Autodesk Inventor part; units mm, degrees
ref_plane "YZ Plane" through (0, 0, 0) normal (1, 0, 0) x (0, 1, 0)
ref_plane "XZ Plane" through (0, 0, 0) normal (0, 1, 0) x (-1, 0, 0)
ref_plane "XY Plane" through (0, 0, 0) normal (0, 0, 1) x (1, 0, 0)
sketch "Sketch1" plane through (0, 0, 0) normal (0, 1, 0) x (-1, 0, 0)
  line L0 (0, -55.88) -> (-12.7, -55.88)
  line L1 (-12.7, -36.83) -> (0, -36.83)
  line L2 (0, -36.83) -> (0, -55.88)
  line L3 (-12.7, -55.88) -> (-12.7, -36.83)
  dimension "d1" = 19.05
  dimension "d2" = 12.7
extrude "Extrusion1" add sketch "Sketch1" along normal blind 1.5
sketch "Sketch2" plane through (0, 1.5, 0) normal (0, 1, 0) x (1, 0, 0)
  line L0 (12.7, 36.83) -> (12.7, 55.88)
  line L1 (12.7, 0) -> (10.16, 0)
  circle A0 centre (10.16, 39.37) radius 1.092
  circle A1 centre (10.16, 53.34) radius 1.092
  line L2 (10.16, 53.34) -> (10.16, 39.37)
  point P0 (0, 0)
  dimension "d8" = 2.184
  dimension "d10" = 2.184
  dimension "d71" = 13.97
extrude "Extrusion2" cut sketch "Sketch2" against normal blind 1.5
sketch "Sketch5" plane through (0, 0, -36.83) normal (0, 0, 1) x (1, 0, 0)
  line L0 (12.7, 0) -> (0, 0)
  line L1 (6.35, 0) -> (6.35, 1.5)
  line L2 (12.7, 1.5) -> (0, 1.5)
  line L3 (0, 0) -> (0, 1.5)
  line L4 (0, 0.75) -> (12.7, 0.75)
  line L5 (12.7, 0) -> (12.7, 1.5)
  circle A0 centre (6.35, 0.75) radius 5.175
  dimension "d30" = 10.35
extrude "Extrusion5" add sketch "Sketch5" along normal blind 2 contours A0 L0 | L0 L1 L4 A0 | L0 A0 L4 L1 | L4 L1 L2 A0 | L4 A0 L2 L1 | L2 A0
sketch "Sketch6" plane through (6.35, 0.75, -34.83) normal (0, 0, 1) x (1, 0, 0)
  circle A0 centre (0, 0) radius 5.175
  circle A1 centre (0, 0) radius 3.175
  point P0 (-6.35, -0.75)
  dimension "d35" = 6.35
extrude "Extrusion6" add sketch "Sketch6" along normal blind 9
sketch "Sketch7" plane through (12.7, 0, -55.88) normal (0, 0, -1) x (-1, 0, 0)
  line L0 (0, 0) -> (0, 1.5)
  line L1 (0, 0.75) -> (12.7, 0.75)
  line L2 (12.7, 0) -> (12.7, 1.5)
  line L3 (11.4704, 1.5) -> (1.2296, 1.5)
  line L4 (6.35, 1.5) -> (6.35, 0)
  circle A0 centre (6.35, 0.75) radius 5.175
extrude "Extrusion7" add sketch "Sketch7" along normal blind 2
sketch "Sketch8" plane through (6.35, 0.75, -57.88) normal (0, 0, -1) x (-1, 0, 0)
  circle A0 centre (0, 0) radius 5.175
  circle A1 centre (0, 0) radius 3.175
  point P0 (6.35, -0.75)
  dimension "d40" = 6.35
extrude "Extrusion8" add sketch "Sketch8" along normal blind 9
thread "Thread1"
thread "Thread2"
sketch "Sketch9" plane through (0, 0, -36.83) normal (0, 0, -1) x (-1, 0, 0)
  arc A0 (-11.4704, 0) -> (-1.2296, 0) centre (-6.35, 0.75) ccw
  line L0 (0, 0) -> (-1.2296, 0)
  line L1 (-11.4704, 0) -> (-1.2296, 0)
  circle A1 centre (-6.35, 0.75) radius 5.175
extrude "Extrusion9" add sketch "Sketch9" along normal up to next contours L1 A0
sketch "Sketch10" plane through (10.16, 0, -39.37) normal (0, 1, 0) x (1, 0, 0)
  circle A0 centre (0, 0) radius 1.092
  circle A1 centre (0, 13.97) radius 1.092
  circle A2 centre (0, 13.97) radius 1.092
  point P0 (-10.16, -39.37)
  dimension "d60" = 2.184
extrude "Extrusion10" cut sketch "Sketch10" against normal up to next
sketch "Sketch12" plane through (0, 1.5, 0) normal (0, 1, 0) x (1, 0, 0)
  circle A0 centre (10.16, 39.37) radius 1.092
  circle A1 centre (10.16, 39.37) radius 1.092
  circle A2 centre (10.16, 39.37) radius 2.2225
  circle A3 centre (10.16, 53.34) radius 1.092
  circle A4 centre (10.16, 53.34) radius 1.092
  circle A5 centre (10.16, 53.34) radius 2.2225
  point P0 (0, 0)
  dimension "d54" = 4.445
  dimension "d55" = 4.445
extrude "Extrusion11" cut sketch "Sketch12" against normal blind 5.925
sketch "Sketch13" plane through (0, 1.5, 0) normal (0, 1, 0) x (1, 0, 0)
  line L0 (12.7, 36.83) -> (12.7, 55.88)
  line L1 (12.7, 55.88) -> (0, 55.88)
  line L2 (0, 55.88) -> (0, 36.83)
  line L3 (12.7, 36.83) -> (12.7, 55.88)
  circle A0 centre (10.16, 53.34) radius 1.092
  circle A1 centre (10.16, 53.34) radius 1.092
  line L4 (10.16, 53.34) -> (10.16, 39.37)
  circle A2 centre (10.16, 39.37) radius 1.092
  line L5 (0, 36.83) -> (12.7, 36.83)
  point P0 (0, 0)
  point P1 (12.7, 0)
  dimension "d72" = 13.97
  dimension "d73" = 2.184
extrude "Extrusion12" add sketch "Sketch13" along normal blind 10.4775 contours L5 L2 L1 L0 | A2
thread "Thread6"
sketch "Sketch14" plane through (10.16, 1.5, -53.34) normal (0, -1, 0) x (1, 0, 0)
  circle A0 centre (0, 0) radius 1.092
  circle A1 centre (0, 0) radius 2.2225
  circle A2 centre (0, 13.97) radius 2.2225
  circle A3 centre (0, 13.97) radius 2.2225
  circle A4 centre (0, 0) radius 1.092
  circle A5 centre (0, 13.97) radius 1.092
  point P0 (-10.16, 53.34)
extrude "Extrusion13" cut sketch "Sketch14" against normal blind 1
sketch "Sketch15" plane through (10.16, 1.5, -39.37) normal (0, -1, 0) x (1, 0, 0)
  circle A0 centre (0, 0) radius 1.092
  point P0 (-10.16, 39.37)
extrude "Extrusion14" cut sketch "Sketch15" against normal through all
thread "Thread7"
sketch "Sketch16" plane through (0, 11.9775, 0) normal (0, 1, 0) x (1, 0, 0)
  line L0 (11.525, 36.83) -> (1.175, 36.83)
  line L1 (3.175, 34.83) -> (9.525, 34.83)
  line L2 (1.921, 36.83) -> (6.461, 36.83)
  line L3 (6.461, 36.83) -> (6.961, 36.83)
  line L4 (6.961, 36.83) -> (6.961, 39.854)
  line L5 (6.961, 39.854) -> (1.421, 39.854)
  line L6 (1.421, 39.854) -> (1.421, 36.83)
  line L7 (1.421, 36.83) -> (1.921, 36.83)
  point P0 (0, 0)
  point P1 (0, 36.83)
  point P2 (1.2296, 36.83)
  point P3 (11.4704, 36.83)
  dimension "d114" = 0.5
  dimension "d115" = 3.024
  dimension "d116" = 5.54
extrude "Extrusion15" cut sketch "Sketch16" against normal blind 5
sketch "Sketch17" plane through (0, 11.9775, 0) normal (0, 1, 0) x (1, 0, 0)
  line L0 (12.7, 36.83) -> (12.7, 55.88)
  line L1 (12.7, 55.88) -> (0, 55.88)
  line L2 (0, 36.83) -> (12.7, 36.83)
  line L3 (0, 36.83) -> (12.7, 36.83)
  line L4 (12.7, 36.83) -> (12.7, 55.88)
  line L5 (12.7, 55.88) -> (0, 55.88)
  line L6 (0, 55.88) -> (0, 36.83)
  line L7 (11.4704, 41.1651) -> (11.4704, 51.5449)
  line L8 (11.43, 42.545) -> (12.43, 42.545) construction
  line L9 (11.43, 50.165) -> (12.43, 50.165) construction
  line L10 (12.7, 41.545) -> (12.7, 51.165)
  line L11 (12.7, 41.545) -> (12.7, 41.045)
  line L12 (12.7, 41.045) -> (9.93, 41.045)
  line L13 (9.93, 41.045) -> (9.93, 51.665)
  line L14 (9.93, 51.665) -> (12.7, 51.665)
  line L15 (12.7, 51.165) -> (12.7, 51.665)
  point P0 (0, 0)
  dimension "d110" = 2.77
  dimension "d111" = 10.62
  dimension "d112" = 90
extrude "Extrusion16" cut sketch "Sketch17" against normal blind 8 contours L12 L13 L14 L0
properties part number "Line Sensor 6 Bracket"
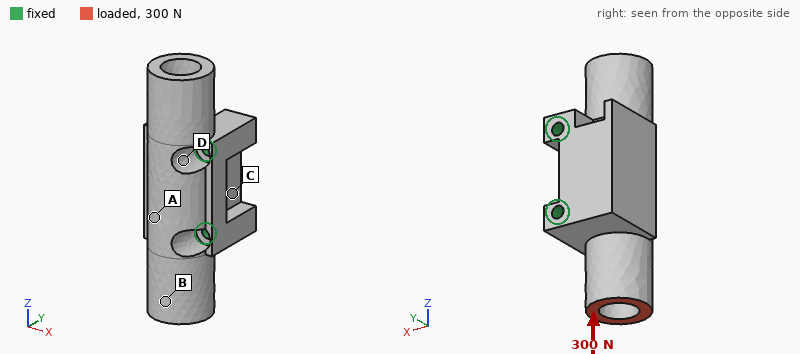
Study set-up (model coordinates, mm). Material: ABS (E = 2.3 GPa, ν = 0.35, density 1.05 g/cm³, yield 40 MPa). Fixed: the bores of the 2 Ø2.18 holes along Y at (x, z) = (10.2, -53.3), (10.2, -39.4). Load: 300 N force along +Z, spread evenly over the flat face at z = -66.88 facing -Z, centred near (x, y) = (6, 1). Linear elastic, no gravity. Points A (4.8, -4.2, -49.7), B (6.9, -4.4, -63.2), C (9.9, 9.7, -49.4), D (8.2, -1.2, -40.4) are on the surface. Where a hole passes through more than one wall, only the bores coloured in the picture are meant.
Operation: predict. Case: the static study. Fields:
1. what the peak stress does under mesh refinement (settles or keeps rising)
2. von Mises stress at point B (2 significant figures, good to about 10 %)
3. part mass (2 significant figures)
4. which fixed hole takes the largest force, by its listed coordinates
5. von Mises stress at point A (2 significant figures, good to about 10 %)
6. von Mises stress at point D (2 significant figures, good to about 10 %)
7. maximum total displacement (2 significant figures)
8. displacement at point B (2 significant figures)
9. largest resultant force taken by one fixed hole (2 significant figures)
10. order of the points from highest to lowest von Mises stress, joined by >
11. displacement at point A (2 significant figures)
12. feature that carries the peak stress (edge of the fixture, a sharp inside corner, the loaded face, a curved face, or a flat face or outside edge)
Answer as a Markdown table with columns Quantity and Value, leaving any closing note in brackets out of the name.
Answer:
| Quantity | Value |
|---|---|
| what the peak stress does under mesh refinement | keeps rising |
| von Mises stress at point B | 5.9 MPa |
| part mass | 4.5 g |
| which fixed hole takes the largest force, by its listed coordinates | (10.2, -53.3) |
| von Mises stress at point A | 4.3 MPa |
| von Mises stress at point D | 2.1 MPa |
| maximum total displacement | 92 µm |
| displacement at point B | 77 µm |
| largest resultant force taken by one fixed hole | 220 N |
| order of the points from highest to lowest von Mises stress, joined by > | B > A > D > C |
| displacement at point A | 29 µm |
| feature that carries the peak stress | edge of the fixture |
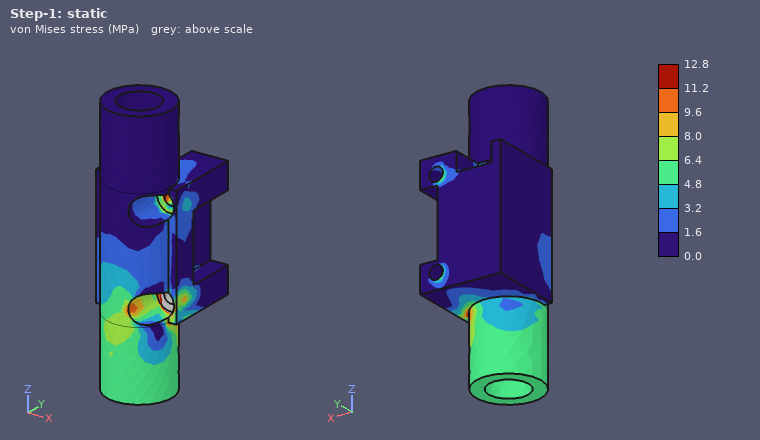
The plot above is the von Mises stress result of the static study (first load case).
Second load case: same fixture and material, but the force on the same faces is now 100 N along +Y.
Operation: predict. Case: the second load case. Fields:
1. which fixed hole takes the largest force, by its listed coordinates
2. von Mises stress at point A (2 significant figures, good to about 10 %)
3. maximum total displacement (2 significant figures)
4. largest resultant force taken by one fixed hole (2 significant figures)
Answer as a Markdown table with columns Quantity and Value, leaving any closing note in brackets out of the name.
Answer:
| Quantity | Value |
|---|---|
| which fixed hole takes the largest force, by its listed coordinates | (10.2, -53.3) |
| von Mises stress at point A | 5.5 MPa |
| maximum total displacement | 0.20 mm |
| largest resultant force taken by one fixed hole | 170 N |
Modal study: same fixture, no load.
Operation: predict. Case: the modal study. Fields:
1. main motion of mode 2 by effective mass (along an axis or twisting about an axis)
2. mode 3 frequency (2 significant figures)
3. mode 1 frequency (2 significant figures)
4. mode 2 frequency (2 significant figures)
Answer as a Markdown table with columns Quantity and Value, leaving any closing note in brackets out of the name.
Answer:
| Quantity | Value |
|---|---|
| main motion of mode 2 by effective mass | twisting about X |
| mode 3 frequency | 7200 Hz |
| mode 1 frequency | 6100 Hz |
| mode 2 frequency | 6400 Hz |
